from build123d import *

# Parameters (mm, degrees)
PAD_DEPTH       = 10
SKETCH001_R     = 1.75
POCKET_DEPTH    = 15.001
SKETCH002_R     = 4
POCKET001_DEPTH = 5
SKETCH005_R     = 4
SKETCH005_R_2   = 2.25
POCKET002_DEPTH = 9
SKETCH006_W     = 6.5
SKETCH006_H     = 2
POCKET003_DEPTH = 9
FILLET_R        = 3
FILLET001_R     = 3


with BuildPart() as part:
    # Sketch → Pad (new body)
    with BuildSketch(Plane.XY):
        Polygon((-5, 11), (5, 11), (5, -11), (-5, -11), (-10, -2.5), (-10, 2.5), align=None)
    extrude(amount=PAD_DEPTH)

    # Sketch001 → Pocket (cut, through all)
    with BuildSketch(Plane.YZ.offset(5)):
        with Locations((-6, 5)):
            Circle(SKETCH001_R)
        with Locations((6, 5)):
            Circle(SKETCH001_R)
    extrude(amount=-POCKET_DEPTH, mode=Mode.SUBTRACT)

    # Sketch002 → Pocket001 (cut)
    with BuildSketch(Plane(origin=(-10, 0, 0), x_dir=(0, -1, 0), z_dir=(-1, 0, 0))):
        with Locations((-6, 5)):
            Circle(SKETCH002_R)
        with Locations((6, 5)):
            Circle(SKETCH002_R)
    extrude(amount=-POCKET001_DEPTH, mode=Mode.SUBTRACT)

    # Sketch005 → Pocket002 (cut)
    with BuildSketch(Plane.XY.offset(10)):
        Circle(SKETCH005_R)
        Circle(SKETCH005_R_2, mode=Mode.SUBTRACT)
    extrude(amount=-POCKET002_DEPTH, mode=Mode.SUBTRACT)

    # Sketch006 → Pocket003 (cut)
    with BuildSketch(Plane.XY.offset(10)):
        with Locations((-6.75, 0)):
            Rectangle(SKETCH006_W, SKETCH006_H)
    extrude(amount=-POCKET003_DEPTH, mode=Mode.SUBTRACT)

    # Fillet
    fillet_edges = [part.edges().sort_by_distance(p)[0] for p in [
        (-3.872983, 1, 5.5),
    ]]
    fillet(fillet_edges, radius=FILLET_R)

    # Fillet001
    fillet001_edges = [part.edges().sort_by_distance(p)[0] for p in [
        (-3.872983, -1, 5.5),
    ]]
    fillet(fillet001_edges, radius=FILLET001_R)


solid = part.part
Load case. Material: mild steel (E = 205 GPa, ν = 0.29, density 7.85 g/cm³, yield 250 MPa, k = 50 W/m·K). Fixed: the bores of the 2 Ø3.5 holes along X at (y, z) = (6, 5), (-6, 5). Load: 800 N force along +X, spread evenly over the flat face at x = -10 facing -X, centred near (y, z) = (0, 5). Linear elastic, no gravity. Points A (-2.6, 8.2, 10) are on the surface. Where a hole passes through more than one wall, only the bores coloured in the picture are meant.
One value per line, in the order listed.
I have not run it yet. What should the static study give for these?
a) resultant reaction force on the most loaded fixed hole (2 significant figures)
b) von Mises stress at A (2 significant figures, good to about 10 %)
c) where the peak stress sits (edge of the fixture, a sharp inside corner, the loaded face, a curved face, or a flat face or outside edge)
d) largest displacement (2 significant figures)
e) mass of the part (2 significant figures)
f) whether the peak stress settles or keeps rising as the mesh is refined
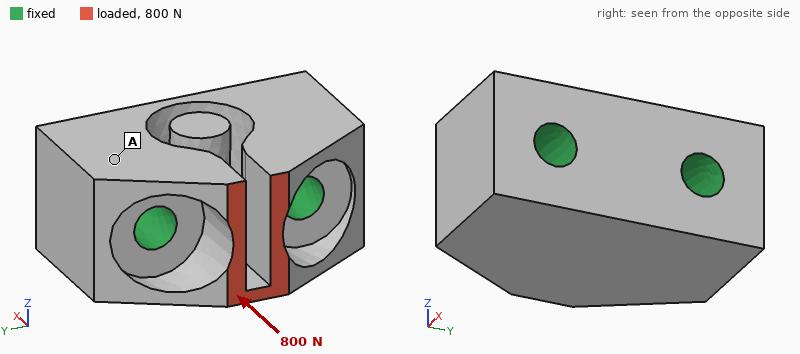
400 N
5.5 MPa
edge of the fixture
3.0 µm
15 g
keeps rising
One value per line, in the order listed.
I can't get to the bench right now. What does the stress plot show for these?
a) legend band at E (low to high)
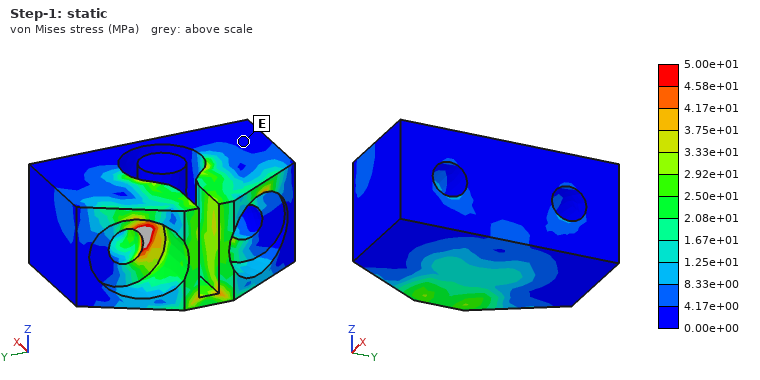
0.00e+00 to 4.17e+00 MPa
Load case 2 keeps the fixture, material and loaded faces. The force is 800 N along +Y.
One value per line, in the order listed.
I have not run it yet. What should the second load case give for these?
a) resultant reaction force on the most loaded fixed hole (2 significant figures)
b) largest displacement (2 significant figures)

440 N
11 µm
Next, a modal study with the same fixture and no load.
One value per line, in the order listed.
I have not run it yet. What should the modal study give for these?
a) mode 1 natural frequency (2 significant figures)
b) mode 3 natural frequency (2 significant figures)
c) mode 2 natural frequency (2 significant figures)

20 kHz
50 kHz
20 kHz
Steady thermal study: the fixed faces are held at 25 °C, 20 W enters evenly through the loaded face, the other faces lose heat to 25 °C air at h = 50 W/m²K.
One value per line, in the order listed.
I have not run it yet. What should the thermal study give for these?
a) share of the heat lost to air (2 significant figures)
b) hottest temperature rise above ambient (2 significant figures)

4.5 %
72 K
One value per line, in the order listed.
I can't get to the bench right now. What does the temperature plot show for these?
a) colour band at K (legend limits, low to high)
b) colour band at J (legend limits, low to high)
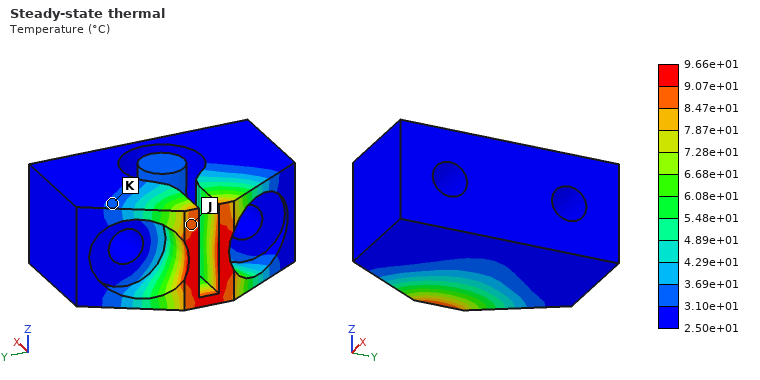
3.10e+01 to 3.69e+01 °C
8.47e+01 to 9.07e+01 °C
